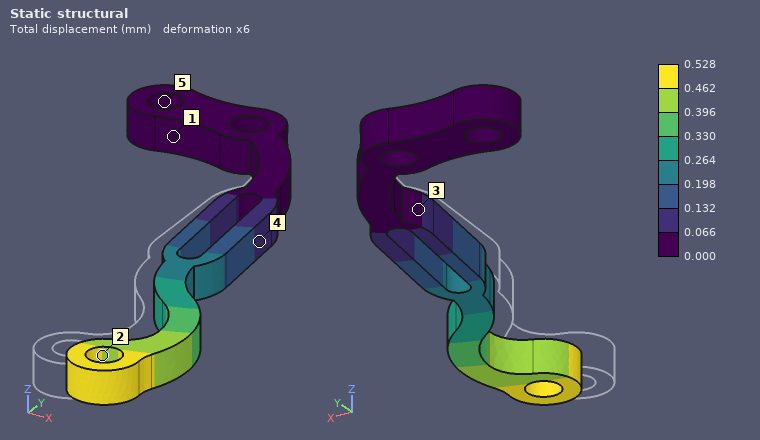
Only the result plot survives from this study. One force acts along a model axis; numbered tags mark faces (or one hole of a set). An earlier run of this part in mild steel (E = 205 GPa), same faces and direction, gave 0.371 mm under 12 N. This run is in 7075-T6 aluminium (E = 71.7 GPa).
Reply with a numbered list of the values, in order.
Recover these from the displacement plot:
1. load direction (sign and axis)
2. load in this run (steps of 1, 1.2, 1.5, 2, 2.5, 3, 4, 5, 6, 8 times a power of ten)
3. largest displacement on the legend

1. +X
2. 6 N
3. 0.528 mm
